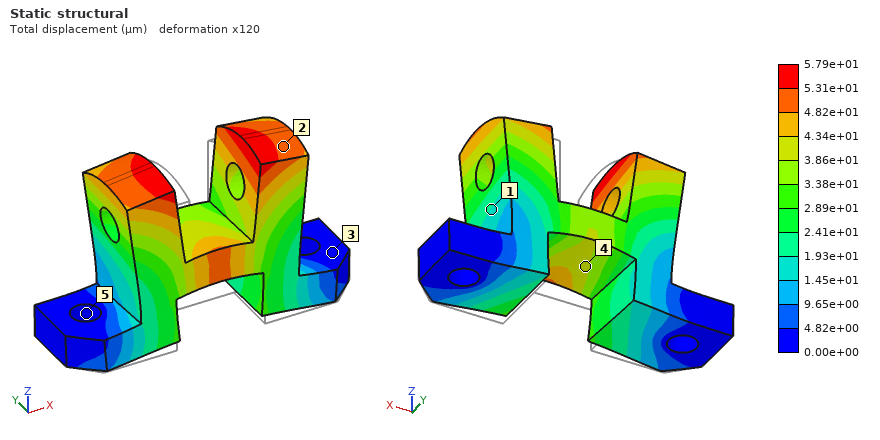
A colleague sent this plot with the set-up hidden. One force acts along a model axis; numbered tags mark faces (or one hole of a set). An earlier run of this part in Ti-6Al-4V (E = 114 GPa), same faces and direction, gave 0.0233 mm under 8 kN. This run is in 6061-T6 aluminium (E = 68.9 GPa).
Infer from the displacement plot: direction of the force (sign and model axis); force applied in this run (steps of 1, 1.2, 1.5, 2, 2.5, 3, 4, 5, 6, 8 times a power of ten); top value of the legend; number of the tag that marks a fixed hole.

+Z
12 kN
5.79e+01 µm
5
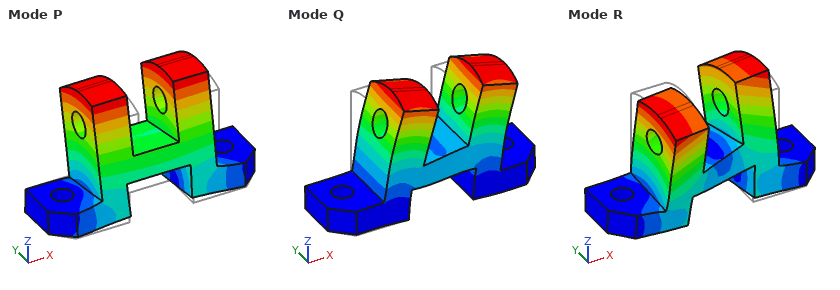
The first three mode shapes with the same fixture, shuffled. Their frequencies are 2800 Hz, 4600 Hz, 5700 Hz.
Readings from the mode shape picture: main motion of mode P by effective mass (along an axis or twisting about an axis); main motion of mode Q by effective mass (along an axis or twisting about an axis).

along Y
along X
